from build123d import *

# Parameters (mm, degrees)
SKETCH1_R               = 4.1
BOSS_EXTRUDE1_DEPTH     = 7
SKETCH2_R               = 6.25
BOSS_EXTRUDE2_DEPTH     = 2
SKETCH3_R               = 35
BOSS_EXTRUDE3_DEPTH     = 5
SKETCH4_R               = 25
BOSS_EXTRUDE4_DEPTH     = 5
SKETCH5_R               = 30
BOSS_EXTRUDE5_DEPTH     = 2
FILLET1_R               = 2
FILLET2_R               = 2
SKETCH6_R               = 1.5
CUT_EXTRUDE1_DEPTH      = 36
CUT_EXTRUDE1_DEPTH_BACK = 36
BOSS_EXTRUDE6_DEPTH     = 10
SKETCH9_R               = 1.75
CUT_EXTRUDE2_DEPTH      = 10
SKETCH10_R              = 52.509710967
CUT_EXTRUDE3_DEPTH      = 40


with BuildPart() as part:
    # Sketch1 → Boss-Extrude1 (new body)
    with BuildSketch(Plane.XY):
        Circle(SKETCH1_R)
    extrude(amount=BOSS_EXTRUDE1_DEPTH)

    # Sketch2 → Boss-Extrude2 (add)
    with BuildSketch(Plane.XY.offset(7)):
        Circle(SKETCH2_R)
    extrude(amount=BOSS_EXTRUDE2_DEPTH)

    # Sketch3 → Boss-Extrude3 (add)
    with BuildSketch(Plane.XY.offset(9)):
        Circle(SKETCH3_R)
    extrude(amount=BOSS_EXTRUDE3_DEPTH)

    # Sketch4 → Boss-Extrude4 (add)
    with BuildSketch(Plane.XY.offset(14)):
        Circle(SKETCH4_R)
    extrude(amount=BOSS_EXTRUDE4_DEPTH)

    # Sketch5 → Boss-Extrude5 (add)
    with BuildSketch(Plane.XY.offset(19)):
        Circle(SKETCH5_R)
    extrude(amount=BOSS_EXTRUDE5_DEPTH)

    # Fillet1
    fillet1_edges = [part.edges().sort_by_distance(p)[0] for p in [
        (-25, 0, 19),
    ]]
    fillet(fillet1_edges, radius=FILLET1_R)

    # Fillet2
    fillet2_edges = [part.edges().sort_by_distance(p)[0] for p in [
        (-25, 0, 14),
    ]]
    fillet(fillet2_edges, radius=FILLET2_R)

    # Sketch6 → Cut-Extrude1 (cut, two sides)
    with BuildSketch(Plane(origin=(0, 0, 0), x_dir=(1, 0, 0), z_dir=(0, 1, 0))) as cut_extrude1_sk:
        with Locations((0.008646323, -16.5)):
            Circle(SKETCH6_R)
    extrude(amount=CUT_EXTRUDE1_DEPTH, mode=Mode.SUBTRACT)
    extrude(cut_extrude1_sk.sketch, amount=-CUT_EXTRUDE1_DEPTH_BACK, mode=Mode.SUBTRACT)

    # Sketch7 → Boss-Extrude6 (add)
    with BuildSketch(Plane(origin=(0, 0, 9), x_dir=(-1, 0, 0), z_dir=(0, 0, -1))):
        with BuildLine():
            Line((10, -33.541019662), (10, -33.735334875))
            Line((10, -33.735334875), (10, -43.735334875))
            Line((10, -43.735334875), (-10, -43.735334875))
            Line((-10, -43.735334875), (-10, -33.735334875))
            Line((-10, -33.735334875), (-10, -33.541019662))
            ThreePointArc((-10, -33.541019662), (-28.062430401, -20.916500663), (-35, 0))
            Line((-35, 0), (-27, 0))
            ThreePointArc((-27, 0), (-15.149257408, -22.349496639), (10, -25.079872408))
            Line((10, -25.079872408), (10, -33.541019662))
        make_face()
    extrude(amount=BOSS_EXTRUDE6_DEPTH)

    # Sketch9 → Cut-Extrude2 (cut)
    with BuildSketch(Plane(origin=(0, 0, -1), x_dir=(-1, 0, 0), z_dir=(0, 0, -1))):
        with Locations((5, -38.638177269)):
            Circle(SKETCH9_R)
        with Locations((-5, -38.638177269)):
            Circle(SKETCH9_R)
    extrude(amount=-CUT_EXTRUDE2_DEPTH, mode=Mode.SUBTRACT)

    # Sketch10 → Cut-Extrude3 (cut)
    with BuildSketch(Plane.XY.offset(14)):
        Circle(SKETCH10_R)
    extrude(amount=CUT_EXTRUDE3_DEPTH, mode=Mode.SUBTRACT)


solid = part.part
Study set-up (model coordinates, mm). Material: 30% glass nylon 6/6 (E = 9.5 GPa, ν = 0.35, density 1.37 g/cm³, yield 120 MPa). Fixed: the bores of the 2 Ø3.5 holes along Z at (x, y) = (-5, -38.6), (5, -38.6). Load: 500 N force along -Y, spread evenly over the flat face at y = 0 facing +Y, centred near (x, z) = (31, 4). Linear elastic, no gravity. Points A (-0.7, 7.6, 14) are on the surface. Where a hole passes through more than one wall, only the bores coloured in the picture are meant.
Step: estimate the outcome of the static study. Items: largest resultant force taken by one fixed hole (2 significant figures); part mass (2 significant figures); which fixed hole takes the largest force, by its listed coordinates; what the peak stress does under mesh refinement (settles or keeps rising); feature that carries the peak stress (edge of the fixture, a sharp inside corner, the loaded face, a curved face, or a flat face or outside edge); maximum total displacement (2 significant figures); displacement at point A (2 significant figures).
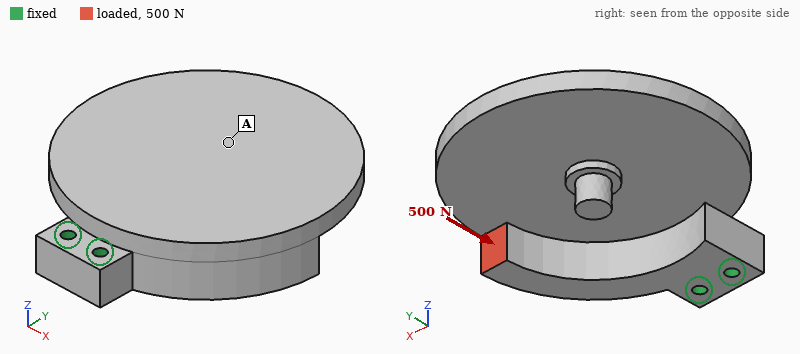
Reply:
1.5 kN
36 g
(5, -38.6)
keeps rising
edge of the fixture
0.42 mm
0.23 mm
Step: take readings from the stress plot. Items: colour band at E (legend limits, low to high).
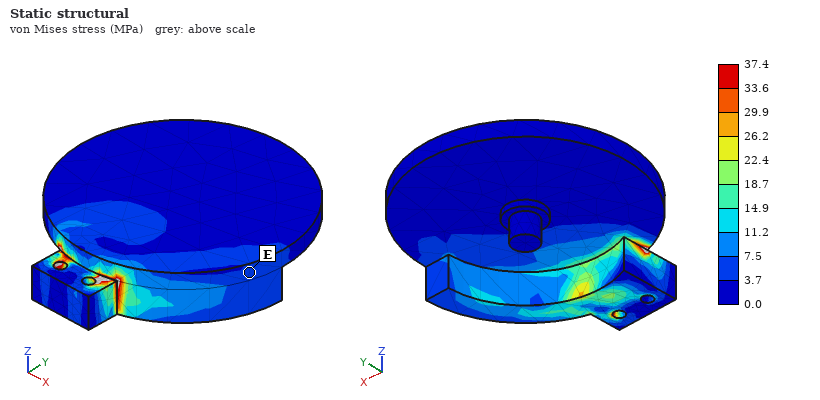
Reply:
3.7 to 7.5 MPa
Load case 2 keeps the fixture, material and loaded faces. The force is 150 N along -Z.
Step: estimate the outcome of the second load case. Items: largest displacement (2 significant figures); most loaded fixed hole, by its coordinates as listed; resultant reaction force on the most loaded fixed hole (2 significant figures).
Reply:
0.50 mm
(5, -38.6)
290 N
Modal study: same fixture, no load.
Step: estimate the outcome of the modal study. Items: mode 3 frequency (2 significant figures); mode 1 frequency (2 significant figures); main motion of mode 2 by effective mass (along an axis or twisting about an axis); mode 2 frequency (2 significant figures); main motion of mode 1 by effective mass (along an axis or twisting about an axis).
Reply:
1400 Hz
550 Hz
along X
1100 Hz
along Z
